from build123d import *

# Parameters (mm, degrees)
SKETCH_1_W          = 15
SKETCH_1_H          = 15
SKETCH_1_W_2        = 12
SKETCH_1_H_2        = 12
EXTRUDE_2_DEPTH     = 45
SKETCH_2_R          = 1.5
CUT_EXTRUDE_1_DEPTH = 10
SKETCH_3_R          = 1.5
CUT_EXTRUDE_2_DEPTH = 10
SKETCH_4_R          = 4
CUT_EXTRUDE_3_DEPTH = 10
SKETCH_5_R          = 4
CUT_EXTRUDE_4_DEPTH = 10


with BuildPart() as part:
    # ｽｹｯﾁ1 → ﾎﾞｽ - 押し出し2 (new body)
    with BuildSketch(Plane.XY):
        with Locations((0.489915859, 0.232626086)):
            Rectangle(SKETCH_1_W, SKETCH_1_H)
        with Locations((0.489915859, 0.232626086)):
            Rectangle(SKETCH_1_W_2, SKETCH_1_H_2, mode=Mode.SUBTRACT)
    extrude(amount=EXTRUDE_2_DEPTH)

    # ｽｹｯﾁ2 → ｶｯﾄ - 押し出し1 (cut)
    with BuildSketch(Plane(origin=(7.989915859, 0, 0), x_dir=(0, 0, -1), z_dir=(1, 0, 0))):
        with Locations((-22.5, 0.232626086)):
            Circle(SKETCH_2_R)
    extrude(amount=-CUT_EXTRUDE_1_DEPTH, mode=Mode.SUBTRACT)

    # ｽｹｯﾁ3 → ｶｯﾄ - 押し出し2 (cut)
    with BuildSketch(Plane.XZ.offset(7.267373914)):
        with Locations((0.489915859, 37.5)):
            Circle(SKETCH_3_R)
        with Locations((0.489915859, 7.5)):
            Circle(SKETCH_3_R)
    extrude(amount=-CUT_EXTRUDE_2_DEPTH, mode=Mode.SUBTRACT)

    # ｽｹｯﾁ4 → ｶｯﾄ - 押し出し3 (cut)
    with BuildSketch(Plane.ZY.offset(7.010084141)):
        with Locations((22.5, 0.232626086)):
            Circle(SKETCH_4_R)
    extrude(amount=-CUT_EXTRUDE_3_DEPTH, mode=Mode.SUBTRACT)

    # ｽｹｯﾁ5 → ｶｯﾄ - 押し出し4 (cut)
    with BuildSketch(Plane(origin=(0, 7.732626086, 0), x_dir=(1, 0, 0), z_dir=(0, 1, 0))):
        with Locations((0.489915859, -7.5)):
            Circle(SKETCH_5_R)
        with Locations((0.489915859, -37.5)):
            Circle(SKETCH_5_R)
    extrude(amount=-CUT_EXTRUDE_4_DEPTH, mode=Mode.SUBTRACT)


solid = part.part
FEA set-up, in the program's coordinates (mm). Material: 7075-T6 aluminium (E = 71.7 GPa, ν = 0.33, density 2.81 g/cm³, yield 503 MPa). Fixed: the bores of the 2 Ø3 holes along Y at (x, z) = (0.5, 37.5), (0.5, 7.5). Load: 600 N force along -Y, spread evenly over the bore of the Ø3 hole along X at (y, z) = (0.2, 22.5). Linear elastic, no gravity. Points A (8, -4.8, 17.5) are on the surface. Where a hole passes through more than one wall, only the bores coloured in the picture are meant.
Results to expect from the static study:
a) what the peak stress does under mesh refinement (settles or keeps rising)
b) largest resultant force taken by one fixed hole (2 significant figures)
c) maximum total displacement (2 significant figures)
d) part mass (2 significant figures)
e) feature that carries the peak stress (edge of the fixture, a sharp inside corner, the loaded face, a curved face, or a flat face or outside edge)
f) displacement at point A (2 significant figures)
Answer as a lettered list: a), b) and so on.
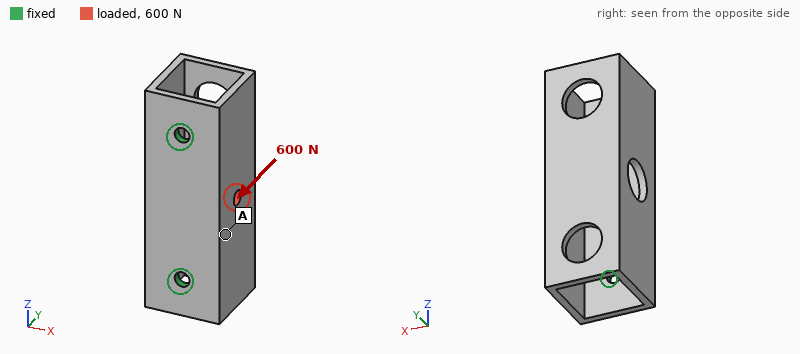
a) keeps rising
b) 320 N
c) 0.15 mm
d) 9.5 g
e) edge of the fixture
f) 0.090 mm
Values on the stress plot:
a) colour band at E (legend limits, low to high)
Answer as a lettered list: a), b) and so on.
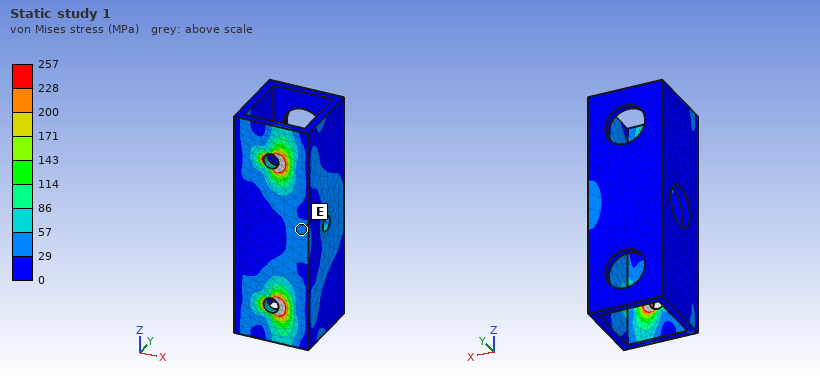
a) 29 to 57 MPa
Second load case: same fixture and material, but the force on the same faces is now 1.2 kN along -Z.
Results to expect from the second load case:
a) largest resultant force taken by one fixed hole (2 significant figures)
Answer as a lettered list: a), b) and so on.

a) 700 N
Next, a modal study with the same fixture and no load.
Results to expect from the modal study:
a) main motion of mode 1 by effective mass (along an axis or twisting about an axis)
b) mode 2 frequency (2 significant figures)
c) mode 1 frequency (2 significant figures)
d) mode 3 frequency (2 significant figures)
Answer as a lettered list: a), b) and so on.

a) along X
b) 8600 Hz
c) 2900 Hz
d) 8900 Hz
